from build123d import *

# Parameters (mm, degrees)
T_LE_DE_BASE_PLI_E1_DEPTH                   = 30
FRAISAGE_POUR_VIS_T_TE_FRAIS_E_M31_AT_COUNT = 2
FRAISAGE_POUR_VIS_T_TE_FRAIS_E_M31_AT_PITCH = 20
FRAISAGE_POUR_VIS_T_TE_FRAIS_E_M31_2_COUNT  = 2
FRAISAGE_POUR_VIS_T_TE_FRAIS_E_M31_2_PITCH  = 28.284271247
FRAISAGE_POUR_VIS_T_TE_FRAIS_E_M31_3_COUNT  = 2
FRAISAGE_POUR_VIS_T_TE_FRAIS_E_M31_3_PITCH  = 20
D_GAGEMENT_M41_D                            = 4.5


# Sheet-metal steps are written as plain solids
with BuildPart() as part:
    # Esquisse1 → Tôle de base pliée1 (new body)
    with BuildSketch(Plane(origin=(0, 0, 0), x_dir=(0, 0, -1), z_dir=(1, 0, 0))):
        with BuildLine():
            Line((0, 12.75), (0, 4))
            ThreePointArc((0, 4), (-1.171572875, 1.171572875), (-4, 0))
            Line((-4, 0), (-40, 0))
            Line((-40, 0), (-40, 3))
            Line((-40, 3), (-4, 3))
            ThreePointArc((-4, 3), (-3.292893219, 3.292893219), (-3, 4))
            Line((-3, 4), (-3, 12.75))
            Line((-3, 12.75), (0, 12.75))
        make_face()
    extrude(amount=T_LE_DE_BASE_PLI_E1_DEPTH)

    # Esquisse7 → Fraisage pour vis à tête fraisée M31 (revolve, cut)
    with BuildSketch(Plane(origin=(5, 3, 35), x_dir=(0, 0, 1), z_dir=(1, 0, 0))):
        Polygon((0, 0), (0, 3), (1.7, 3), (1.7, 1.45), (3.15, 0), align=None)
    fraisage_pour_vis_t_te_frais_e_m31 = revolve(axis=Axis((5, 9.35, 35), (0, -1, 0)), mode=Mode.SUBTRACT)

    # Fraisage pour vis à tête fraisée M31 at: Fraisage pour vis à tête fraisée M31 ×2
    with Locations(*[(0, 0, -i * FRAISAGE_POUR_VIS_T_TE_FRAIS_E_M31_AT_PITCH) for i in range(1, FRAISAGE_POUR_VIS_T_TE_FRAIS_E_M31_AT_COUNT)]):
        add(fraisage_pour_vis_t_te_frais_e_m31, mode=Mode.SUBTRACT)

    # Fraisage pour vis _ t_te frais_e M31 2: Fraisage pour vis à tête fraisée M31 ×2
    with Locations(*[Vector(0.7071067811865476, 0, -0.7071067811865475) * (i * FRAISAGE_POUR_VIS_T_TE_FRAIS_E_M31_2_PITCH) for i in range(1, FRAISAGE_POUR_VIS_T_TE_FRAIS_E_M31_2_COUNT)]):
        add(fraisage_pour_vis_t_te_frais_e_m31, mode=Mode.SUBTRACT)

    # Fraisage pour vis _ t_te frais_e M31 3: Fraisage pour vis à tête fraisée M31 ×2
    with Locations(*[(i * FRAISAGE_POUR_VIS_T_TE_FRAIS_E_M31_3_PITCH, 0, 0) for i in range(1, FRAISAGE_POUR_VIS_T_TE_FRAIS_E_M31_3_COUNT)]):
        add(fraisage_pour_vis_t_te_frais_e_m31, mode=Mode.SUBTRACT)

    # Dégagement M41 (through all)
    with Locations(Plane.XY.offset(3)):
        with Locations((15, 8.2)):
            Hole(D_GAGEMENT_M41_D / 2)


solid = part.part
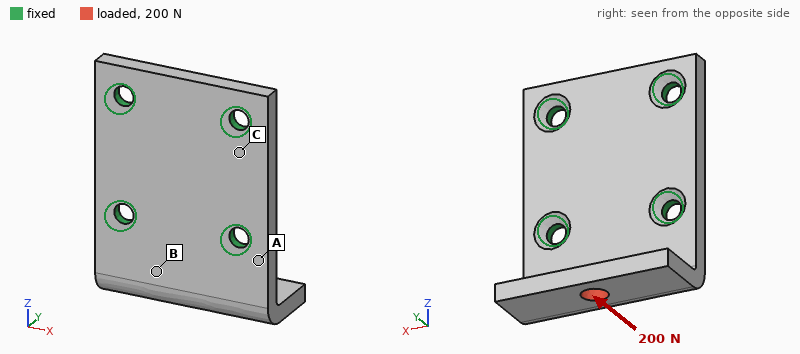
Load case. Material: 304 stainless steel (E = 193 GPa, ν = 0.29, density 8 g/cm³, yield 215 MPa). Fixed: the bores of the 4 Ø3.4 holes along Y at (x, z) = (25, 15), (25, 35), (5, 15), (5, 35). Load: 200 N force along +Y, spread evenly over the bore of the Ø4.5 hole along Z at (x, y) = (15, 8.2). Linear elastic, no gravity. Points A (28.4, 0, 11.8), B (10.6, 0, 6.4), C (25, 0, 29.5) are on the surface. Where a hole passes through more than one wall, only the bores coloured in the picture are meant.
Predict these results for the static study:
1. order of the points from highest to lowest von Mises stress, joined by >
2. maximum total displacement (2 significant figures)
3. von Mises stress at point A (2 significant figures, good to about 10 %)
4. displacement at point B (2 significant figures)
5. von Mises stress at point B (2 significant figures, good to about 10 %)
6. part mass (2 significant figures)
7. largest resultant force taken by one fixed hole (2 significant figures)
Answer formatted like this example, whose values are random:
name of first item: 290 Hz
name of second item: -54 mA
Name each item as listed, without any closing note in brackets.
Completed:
order of the points from highest to lowest von Mises stress, joined by >: A > B > C
maximum total displacement: 29 µm
von Mises stress at point A: 55 MPa
displacement at point B: 10.0 µm
von Mises stress at point B: 20 MPa
part mass: 33 g
largest resultant force taken by one fixed hole: 150 N
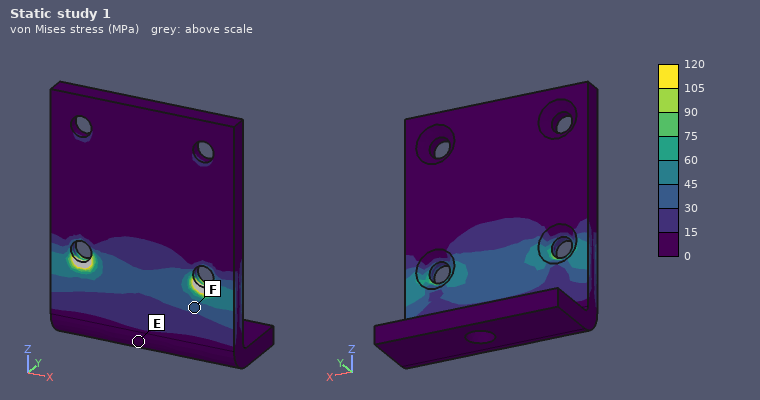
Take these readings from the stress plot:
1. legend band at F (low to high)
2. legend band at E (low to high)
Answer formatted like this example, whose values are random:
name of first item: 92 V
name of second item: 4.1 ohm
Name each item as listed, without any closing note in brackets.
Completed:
legend band at F: 30 to 45 MPa
legend band at E: 0 to 15 MPa
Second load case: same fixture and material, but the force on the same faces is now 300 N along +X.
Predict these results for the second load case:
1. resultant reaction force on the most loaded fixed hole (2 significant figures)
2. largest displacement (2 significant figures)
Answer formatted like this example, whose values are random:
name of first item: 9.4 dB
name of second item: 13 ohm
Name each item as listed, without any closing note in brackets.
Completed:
resultant reaction force on the most loaded fixed hole: 260 N
largest displacement: 13 µm
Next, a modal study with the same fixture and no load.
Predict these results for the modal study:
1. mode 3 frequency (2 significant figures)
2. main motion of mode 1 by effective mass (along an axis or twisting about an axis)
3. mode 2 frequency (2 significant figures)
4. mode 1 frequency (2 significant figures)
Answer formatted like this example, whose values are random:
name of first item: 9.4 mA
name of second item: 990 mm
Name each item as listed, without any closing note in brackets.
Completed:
mode 3 frequency: 15 kHz
main motion of mode 1 by effective mass: along Y
mode 2 frequency: 8200 Hz
mode 1 frequency: 4600 Hz
